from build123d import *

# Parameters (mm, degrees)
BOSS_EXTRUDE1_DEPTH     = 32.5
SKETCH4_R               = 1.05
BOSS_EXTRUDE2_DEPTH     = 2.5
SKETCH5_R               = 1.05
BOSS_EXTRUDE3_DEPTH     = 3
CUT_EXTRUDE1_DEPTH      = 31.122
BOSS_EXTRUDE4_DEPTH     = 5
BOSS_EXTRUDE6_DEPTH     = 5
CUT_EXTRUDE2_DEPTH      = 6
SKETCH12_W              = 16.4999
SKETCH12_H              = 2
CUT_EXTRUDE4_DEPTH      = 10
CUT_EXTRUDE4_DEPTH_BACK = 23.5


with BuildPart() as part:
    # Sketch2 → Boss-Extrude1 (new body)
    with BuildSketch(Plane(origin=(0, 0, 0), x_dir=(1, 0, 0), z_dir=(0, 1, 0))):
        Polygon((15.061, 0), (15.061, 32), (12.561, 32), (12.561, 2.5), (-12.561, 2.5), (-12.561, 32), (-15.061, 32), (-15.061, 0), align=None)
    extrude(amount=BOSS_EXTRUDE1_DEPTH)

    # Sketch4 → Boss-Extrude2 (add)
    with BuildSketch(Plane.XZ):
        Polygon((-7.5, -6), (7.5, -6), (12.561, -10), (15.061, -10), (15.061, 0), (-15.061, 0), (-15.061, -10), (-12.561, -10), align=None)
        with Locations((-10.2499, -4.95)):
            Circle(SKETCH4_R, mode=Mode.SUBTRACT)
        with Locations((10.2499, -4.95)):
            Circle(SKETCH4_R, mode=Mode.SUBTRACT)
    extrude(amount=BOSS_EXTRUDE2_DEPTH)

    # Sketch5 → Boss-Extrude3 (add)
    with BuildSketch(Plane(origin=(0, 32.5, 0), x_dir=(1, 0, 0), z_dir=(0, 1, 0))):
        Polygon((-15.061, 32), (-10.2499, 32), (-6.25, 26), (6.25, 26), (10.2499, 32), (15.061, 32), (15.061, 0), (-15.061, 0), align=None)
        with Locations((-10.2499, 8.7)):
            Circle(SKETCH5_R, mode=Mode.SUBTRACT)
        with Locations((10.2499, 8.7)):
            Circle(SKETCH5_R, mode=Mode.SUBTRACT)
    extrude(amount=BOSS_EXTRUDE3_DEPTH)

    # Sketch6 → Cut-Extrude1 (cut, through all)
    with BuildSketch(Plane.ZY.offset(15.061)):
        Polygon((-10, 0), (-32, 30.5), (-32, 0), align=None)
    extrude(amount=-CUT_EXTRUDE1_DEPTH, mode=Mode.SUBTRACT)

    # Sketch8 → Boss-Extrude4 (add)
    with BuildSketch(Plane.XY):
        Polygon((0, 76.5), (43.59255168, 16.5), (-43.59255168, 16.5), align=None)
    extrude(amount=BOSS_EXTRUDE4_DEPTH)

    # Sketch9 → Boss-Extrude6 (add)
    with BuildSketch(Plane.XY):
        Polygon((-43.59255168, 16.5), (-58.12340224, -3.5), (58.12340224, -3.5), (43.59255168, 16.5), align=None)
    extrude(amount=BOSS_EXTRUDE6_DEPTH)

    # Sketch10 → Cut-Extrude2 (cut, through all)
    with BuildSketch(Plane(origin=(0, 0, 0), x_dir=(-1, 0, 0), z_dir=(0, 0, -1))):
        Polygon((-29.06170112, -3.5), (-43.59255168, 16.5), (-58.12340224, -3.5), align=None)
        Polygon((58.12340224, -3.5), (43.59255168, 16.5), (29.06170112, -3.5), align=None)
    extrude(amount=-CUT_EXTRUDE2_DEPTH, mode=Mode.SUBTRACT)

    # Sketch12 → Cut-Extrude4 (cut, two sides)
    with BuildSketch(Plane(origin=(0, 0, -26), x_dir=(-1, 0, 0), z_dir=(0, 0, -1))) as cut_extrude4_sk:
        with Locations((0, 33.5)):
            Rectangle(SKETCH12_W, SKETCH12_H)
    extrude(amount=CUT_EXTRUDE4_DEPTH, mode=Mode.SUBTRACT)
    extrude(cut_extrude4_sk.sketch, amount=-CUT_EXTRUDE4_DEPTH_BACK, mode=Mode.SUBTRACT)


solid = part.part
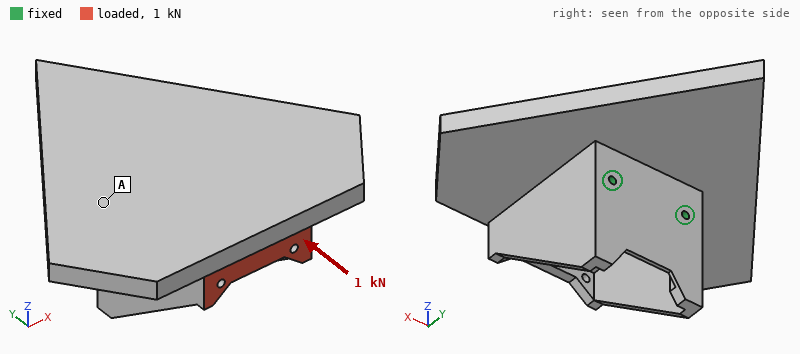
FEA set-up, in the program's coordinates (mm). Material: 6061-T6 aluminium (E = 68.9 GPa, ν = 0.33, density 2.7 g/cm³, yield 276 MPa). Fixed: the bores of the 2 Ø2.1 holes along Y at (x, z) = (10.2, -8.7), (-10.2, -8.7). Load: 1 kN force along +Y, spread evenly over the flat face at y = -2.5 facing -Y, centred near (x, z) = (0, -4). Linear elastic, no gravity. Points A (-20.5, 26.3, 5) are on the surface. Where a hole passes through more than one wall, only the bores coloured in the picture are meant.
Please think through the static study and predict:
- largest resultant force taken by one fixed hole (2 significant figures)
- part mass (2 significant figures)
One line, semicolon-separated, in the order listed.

500 N; 76 g
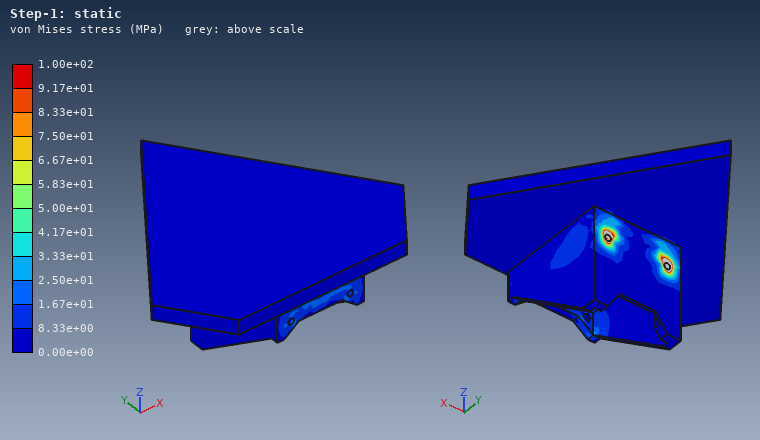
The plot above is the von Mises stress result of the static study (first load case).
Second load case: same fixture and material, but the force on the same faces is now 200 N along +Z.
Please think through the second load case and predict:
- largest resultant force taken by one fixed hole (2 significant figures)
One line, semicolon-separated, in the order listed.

100 N
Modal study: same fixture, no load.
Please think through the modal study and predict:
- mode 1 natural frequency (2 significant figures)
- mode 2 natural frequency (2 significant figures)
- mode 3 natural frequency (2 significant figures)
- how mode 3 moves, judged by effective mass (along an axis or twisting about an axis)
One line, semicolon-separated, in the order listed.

1000 Hz; 2400 Hz; 3900 Hz; along X
